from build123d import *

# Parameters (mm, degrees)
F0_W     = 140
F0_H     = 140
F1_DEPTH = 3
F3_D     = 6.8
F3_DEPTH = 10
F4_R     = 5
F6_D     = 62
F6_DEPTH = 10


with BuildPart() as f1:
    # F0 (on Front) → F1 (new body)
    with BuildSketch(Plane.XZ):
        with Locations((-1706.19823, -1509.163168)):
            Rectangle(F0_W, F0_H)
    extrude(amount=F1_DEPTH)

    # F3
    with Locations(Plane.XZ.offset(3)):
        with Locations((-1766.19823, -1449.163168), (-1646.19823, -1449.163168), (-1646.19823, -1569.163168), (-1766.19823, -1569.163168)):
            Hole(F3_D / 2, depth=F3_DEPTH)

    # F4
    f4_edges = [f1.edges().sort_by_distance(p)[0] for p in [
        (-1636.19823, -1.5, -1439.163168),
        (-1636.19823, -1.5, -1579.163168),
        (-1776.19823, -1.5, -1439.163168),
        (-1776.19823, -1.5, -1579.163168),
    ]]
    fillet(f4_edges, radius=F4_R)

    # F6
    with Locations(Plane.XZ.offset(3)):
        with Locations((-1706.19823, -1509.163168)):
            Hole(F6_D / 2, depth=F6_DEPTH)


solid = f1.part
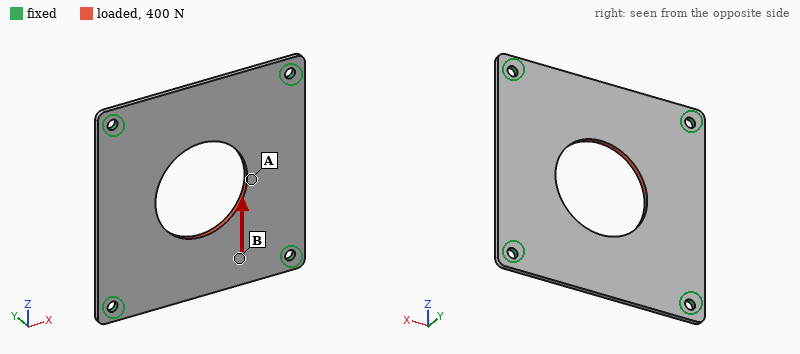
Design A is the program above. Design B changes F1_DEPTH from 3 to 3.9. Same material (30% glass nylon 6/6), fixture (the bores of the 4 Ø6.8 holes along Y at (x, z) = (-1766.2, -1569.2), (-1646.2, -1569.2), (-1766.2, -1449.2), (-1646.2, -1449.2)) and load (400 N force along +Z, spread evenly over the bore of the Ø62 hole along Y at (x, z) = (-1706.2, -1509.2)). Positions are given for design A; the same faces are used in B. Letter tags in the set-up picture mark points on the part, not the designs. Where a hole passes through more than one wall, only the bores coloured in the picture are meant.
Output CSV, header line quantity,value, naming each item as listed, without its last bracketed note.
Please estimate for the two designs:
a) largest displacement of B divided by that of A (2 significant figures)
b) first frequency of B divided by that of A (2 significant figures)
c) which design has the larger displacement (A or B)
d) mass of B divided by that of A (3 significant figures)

quantity,value
largest displacement of B divided by that of A,0.77
first frequency of B divided by that of A,1.3
which design has the larger displacement,A
mass of B divided by that of A,1.30
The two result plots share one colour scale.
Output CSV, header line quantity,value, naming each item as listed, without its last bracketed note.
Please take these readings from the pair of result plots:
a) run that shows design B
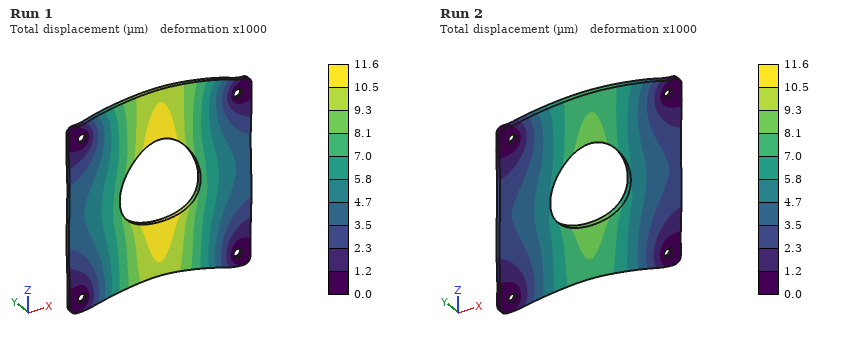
quantity,value
run that shows design B,Run 2
